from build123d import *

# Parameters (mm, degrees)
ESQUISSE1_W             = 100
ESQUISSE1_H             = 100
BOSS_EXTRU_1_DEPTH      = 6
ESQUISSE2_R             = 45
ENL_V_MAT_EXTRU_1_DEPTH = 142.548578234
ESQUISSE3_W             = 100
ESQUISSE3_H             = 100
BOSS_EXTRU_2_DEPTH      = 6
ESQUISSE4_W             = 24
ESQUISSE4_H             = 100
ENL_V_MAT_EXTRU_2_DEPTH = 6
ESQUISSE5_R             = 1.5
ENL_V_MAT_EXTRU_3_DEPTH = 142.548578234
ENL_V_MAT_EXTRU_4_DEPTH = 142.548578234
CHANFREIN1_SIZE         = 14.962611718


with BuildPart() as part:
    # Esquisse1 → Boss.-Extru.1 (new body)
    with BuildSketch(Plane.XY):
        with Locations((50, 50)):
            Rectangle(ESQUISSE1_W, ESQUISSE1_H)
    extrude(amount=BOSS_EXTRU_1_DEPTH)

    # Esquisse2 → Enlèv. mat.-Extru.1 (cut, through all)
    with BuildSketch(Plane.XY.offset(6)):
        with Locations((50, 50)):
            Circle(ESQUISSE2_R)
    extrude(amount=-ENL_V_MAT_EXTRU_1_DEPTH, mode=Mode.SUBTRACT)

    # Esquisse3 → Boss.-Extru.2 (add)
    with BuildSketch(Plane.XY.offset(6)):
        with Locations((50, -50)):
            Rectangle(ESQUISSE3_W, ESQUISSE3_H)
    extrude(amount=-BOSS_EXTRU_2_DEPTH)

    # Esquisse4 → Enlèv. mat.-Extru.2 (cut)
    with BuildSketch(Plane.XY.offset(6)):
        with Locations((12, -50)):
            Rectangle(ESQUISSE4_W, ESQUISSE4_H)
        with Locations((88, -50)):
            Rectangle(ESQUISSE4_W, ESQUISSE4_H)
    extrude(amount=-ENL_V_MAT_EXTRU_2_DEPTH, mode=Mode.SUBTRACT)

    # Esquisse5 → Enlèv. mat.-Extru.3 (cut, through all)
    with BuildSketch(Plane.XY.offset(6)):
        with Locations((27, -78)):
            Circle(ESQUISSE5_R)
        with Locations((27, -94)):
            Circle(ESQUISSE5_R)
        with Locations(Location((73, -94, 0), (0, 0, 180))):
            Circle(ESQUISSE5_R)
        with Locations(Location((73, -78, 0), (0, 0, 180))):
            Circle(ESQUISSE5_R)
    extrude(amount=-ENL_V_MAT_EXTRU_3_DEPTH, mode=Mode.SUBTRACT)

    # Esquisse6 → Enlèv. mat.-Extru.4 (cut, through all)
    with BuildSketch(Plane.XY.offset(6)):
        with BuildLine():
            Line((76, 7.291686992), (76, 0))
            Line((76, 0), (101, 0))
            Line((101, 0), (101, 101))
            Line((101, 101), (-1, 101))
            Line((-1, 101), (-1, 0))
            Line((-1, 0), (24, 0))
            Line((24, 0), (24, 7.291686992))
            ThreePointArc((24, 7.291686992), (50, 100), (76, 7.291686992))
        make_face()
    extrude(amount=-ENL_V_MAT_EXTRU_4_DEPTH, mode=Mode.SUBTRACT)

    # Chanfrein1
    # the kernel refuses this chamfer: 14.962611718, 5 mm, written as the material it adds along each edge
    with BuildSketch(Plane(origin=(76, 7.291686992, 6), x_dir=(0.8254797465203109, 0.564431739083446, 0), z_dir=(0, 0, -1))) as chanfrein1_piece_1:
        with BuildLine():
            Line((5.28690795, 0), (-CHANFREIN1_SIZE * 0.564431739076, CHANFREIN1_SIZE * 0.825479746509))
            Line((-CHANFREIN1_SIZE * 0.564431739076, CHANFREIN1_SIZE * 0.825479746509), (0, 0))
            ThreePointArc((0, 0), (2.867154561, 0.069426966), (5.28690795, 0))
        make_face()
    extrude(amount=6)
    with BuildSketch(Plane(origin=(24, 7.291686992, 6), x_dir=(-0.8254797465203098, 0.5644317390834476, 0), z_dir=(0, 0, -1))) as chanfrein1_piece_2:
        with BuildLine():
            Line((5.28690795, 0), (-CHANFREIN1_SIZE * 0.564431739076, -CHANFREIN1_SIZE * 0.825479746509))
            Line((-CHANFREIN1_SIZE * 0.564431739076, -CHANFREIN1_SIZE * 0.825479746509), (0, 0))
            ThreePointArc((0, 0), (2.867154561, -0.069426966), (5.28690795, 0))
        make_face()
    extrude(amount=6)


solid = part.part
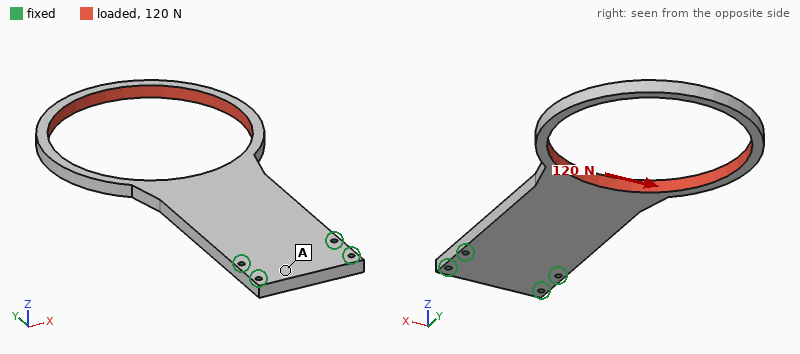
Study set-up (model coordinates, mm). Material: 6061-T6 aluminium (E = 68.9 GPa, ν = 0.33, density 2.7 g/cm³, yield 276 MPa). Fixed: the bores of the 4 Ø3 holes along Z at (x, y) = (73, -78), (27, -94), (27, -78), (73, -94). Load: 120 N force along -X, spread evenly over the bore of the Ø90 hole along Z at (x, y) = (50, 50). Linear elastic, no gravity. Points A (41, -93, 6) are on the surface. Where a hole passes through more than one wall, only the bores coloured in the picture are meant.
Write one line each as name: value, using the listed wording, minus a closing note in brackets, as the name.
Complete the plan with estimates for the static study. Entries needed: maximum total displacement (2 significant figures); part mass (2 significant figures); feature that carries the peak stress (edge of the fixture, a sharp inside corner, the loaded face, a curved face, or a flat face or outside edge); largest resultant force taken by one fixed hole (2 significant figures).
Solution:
maximum total displacement: 0.52 mm
part mass: 110 g
feature that carries the peak stress: the loaded face
largest resultant force taken by one fixed hole: 300 N
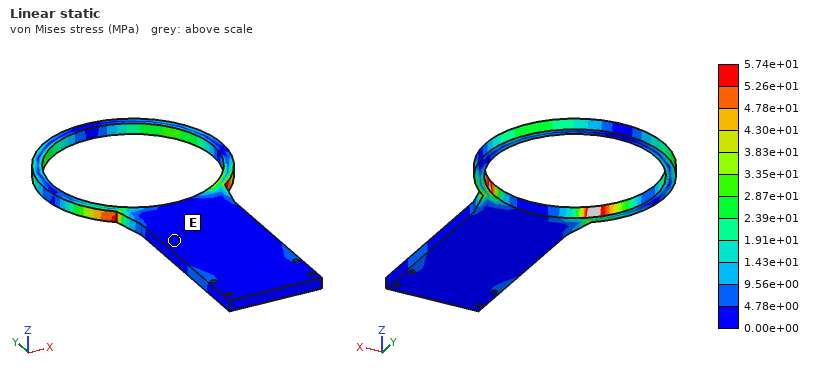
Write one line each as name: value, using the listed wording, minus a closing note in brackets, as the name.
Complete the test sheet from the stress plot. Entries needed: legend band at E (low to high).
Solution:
legend band at E: 0.00e+00 to 4.78e+00 MPa
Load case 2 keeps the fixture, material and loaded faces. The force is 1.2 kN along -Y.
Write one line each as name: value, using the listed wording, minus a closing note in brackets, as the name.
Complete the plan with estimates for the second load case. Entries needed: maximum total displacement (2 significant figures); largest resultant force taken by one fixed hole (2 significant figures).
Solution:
maximum total displacement: 0.66 mm
largest resultant force taken by one fixed hole: 460 N
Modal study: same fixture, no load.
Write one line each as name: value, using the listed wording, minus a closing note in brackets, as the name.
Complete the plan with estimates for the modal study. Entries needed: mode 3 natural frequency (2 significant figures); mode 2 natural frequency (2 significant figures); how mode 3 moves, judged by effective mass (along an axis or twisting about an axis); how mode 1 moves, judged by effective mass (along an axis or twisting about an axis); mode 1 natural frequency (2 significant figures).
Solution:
mode 3 natural frequency: 640 Hz
mode 2 natural frequency: 530 Hz
how mode 3 moves, judged by effective mass: twisting about Y
how mode 1 moves, judged by effective mass: along Z
mode 1 natural frequency: 220 Hz
